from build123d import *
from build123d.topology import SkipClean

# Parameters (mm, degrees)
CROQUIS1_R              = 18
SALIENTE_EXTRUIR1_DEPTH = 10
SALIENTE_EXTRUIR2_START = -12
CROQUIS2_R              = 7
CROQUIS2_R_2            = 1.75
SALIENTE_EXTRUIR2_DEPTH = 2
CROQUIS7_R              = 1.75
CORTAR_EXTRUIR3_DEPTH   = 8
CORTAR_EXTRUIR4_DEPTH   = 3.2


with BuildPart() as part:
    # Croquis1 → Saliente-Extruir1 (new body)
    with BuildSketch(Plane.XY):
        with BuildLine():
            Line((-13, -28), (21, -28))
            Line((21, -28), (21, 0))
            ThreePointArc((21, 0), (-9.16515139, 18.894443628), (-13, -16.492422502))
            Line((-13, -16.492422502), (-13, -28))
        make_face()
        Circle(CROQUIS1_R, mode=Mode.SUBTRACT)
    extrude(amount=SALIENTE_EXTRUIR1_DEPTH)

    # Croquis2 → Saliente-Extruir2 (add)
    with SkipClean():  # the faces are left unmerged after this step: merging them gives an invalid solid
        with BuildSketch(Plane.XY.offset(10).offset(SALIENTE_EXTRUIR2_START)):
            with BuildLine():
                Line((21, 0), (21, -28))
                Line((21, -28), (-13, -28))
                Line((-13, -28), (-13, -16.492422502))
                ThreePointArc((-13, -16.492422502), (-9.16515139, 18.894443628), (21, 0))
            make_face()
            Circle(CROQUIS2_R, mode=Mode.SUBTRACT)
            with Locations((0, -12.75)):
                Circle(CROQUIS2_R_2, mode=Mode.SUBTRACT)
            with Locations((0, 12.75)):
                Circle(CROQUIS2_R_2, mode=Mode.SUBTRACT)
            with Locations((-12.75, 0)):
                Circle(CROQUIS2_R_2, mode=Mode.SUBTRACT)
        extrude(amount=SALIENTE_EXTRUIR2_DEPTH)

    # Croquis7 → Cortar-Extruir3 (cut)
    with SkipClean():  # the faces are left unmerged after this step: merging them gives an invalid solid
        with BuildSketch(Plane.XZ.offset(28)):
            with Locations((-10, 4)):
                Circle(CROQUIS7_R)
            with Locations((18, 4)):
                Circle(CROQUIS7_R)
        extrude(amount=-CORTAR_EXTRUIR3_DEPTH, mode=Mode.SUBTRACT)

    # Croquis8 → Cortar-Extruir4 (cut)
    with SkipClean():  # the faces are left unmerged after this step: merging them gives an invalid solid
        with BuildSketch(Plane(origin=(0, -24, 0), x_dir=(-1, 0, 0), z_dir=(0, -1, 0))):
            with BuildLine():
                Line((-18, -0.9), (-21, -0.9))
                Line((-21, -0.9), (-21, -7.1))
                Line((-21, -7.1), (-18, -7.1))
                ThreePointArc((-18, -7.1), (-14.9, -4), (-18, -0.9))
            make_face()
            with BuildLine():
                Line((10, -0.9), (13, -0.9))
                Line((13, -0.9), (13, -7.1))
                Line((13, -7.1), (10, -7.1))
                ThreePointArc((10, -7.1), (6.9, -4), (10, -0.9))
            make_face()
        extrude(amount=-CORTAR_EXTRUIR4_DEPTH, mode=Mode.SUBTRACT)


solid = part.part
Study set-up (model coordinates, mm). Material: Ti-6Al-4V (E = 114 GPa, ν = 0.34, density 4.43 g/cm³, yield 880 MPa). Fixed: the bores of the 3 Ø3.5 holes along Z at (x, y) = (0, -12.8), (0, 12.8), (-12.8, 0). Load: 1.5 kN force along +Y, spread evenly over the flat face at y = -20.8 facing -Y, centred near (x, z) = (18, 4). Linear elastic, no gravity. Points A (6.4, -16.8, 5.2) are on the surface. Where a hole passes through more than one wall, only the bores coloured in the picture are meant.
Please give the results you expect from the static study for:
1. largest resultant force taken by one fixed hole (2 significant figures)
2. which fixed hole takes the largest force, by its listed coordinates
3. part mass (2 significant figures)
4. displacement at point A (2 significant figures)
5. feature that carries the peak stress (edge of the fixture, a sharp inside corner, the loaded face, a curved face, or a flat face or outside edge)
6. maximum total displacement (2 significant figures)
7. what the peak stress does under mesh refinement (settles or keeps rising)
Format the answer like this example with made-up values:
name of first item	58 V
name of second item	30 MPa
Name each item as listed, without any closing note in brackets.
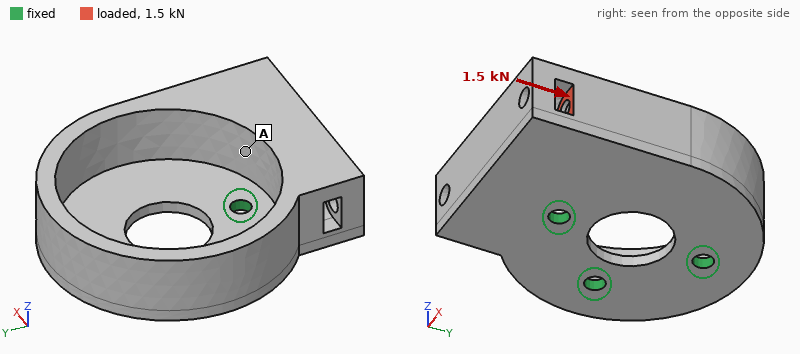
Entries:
largest resultant force taken by one fixed hole	1.3 kN
which fixed hole takes the largest force, by its listed coordinates	(0, -12.8)
part mass	44 g
displacement at point A	17 µm
feature that carries the peak stress	edge of the fixture
maximum total displacement	43 µm
what the peak stress does under mesh refinement	keeps rising
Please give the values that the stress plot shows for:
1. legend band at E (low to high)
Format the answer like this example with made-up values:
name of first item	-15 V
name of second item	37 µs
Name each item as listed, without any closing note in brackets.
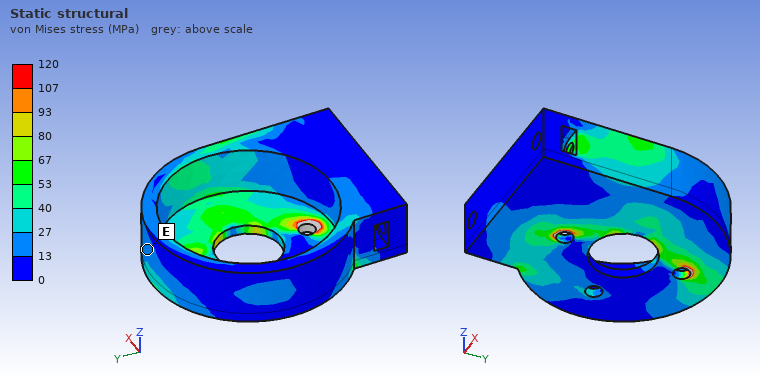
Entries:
legend band at E	13 to 27 MPa
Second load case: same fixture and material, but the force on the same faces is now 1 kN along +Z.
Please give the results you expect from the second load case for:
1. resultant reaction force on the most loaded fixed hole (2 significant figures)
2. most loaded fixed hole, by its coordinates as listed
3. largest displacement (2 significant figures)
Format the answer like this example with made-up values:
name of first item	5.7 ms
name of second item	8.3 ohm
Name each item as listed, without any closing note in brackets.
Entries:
resultant reaction force on the most loaded fixed hole	1.7 kN
most loaded fixed hole, by its coordinates as listed	(0, -12.8)
largest displacement	0.15 mm
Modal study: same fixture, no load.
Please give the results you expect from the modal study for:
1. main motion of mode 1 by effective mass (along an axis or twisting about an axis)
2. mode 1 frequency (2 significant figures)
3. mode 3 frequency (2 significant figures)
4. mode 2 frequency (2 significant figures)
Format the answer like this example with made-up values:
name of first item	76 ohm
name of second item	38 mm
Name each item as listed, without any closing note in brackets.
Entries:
main motion of mode 1 by effective mass	along Z
mode 1 frequency	4000 Hz
mode 3 frequency	9500 Hz
mode 2 frequency	5600 Hz
